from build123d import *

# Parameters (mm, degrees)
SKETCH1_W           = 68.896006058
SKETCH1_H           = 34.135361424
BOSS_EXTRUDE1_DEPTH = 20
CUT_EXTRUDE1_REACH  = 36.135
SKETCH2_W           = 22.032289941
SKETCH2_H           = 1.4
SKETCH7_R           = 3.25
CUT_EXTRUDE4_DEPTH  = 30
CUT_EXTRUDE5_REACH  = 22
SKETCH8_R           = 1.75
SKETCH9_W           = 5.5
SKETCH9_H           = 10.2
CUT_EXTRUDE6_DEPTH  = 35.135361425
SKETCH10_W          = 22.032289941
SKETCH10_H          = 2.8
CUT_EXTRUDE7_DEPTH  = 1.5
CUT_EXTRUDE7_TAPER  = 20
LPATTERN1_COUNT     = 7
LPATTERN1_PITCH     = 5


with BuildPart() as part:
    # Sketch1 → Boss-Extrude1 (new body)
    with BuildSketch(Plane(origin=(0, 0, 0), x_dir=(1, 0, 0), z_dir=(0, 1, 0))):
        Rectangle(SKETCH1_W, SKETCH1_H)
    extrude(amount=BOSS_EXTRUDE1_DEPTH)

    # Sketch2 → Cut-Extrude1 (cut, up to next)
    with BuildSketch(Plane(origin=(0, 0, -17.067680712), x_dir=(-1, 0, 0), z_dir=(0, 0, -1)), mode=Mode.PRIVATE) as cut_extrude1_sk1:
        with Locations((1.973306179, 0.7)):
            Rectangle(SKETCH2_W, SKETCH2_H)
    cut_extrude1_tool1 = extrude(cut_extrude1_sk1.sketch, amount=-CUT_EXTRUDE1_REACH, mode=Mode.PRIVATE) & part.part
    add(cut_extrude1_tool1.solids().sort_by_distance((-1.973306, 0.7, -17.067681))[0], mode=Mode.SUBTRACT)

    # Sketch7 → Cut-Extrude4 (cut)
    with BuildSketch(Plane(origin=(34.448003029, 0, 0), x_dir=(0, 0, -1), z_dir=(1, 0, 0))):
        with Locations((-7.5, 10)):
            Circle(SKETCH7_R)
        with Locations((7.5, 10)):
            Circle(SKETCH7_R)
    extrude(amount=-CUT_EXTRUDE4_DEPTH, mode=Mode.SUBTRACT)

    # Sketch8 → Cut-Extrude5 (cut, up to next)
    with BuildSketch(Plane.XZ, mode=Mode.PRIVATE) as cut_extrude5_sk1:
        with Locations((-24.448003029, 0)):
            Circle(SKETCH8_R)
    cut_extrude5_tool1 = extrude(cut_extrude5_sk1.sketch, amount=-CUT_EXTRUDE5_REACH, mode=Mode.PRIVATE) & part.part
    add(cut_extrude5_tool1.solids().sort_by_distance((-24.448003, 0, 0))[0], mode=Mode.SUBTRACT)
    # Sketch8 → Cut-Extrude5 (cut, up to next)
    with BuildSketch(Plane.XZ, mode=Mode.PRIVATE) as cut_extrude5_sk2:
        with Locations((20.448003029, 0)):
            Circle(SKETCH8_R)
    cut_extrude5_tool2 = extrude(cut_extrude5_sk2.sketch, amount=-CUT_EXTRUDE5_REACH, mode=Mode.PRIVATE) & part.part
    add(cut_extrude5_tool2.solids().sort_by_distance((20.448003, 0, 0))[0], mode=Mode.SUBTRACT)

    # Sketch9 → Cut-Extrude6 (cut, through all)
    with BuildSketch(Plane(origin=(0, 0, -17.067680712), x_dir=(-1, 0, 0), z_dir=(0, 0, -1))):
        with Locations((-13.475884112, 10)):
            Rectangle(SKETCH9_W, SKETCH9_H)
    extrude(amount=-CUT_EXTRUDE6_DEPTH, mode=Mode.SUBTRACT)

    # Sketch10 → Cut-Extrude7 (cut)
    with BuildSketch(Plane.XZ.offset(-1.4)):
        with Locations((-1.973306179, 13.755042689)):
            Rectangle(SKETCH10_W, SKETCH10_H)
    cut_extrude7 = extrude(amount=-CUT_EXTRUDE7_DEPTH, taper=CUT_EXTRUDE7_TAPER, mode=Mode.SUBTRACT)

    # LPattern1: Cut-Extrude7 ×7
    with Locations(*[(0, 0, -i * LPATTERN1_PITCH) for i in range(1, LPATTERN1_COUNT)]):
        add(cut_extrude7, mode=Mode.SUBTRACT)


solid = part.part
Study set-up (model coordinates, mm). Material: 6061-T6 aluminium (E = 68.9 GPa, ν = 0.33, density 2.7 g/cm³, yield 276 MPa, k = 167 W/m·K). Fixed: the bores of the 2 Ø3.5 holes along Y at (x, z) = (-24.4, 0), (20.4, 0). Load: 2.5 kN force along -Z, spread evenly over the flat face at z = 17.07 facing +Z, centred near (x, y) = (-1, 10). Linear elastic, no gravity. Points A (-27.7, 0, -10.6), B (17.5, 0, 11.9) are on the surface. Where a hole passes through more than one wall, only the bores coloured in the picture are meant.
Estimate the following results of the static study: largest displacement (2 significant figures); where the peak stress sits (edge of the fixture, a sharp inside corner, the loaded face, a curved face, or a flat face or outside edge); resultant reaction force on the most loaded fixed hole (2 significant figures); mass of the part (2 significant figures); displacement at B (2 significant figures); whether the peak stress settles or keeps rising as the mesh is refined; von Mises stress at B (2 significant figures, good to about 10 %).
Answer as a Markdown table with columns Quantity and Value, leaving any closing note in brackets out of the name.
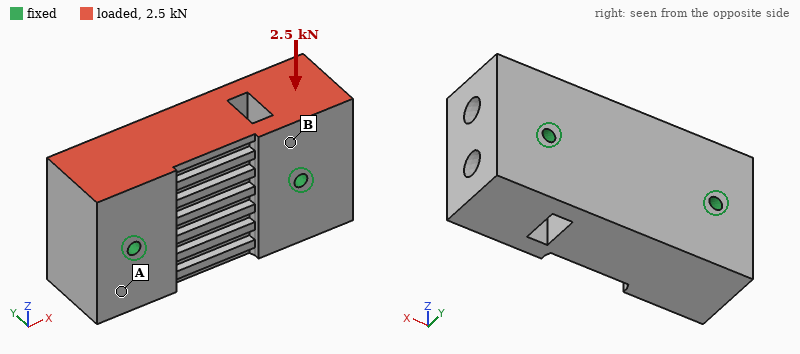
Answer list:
| Quantity | Value |
|---|---|
| largest displacement | 1.8 µm |
| where the peak stress sits | edge of the fixture |
| resultant reaction force on the most loaded fixed hole | 1.3 kN |
| mass of the part | 110 g |
| displacement at B | 0.75 µm |
| whether the peak stress settles or keeps rising as the mesh is refined | keeps rising |
| von Mises stress at B | 2.8 MPa |
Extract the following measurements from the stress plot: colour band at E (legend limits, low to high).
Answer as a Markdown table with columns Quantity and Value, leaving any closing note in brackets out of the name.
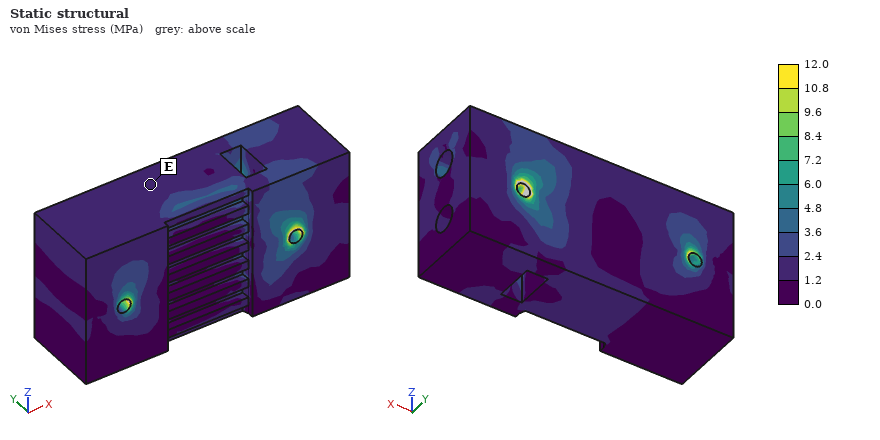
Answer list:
| Quantity | Value |
|---|---|
| colour band at E | 1.2 to 2.4 MPa |
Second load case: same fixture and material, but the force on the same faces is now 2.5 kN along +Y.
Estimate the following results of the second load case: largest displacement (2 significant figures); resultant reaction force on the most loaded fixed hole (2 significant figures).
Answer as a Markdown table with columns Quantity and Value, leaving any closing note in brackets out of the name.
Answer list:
| Quantity | Value |
|---|---|
| largest displacement | 9.8 µm |
| resultant reaction force on the most loaded fixed hole | 1.3 kN |
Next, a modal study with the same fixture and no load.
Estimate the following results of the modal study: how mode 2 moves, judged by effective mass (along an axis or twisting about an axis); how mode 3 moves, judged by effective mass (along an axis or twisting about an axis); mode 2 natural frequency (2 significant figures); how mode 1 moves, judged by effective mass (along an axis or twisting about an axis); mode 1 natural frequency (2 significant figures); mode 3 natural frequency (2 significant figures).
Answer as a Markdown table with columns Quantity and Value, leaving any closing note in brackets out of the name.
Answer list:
| Quantity | Value |
|---|---|
| how mode 2 moves, judged by effective mass | twisting about X |
| how mode 3 moves, judged by effective mass | along Z |
| mode 2 natural frequency | 17 kHz |
| how mode 1 moves, judged by effective mass | along Y |
| mode 1 natural frequency | 17 kHz |
| mode 3 natural frequency | 20 kHz |
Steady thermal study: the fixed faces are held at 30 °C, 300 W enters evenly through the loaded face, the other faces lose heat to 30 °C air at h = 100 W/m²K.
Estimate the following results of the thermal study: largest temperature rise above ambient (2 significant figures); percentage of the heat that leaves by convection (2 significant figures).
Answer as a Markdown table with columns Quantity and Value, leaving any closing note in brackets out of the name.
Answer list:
| Quantity | Value |
|---|---|
| largest temperature rise above ambient | 41 K |
| percentage of the heat that leaves by convection | 5.0 % |
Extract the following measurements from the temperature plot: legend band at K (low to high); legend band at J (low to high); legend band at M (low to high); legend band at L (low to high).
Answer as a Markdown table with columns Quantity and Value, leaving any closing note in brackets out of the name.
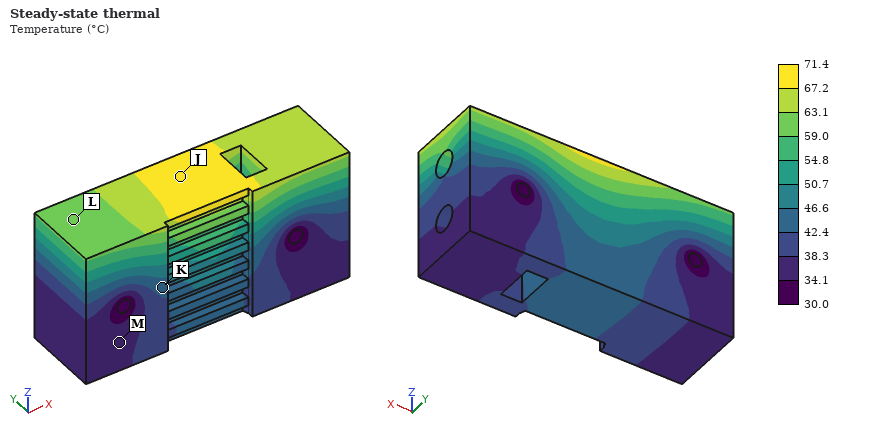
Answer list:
| Quantity | Value |
|---|---|
| legend band at K | 42.4 to 46.6 °C |
| legend band at J | 67.2 to 71.4 °C |
| legend band at M | 34.1 to 38.3 °C |
| legend band at L | 59.0 to 63.1 °C |
